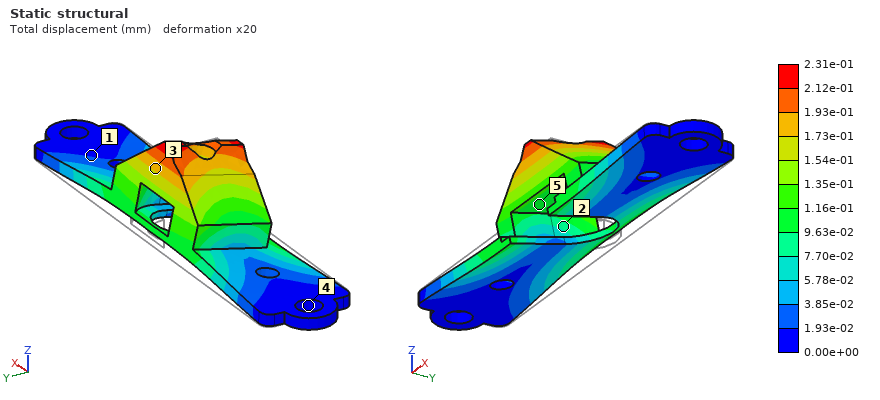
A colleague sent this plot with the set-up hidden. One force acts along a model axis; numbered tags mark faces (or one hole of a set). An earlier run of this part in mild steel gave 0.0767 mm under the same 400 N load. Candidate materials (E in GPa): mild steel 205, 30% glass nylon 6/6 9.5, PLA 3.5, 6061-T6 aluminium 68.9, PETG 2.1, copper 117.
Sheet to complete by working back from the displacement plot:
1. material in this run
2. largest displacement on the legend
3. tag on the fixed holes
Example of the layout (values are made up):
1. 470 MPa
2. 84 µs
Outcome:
1. 6061-T6 aluminium
2. 2.31e-01 mm
3. 4
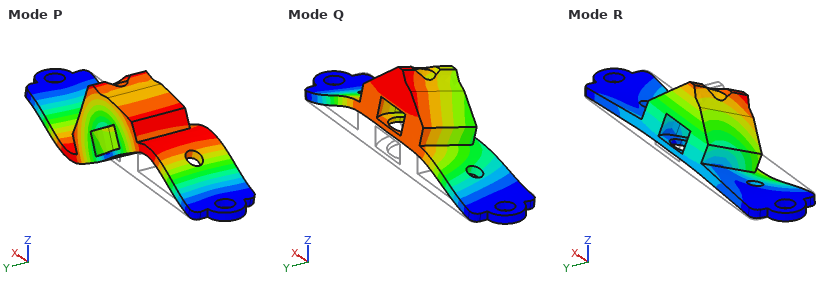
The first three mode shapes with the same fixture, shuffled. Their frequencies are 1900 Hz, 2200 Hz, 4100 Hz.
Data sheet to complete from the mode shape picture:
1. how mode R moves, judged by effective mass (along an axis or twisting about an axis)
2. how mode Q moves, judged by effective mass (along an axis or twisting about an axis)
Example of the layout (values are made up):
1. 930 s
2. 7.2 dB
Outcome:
1. along Y
2. along Z
